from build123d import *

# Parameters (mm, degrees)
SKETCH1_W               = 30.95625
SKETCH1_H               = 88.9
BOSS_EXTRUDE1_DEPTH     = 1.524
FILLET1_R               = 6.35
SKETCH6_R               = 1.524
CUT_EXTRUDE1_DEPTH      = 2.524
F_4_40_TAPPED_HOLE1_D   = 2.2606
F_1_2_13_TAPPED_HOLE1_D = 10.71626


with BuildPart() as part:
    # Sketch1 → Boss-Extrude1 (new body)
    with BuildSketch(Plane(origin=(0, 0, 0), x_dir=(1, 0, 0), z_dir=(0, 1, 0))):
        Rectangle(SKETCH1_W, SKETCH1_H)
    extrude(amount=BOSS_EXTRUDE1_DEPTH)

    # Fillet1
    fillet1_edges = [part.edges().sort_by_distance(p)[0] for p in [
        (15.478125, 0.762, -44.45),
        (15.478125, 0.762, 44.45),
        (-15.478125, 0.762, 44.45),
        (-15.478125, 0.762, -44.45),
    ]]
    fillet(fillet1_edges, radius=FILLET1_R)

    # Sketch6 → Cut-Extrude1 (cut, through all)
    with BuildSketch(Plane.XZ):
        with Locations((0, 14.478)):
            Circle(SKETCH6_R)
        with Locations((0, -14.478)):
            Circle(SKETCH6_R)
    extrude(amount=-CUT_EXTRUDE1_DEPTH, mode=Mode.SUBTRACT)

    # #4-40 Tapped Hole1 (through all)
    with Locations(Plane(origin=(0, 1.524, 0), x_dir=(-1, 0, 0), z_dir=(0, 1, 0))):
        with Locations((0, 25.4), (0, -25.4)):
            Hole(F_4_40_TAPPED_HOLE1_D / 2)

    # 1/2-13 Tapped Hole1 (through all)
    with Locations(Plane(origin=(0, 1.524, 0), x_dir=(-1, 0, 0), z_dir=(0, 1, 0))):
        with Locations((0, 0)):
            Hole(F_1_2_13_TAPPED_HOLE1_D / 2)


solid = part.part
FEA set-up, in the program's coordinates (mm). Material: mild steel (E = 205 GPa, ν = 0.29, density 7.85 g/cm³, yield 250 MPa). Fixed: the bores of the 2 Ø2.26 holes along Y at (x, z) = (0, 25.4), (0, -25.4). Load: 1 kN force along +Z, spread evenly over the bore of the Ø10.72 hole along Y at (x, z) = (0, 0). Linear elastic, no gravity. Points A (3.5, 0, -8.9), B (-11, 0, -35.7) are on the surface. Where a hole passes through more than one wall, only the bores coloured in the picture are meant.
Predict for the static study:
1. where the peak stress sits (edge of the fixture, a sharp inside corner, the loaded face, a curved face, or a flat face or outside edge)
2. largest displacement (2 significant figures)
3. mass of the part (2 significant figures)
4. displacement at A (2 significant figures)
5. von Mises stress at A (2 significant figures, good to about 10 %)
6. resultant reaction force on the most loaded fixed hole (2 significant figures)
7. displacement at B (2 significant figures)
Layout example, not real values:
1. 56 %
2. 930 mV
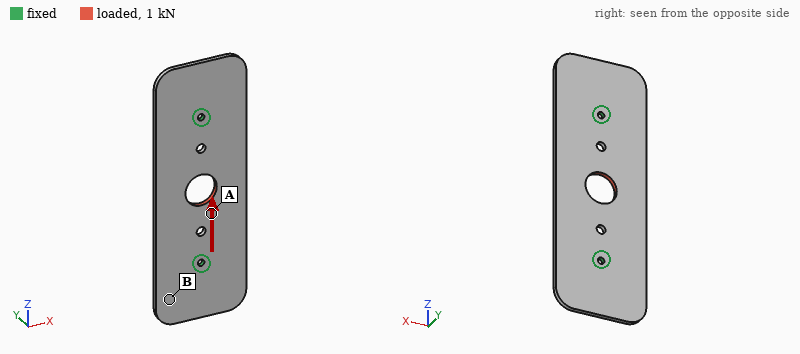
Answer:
1. edge of the fixture
2. 2.5 µm
3. 31 g
4. 2.0 µm
5. 21 MPa
6. 500 N
7. 0.92 µm
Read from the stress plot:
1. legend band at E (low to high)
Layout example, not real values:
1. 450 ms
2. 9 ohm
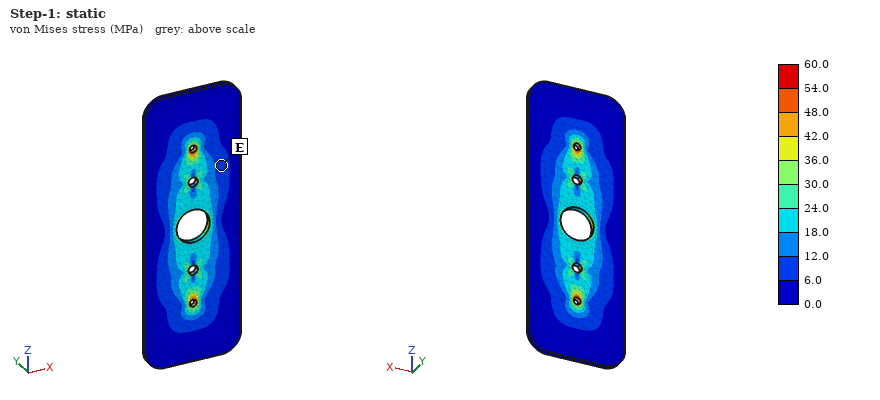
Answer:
1. 6.0 to 12.0 MPa
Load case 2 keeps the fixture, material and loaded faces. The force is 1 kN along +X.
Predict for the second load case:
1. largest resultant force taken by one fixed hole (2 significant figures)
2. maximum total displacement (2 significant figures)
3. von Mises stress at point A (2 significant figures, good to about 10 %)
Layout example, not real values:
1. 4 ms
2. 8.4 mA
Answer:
1. 500 N
2. 7.7 µm
3. 23 MPa
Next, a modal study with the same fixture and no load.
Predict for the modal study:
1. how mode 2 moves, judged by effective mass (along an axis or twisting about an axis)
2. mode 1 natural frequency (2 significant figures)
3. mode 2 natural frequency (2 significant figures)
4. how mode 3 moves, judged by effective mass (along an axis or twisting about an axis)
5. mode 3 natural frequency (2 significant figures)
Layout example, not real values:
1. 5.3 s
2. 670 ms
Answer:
1. twisting about Z
2. 2300 Hz
3. 2600 Hz
4. twisting about X
5. 3000 Hz
